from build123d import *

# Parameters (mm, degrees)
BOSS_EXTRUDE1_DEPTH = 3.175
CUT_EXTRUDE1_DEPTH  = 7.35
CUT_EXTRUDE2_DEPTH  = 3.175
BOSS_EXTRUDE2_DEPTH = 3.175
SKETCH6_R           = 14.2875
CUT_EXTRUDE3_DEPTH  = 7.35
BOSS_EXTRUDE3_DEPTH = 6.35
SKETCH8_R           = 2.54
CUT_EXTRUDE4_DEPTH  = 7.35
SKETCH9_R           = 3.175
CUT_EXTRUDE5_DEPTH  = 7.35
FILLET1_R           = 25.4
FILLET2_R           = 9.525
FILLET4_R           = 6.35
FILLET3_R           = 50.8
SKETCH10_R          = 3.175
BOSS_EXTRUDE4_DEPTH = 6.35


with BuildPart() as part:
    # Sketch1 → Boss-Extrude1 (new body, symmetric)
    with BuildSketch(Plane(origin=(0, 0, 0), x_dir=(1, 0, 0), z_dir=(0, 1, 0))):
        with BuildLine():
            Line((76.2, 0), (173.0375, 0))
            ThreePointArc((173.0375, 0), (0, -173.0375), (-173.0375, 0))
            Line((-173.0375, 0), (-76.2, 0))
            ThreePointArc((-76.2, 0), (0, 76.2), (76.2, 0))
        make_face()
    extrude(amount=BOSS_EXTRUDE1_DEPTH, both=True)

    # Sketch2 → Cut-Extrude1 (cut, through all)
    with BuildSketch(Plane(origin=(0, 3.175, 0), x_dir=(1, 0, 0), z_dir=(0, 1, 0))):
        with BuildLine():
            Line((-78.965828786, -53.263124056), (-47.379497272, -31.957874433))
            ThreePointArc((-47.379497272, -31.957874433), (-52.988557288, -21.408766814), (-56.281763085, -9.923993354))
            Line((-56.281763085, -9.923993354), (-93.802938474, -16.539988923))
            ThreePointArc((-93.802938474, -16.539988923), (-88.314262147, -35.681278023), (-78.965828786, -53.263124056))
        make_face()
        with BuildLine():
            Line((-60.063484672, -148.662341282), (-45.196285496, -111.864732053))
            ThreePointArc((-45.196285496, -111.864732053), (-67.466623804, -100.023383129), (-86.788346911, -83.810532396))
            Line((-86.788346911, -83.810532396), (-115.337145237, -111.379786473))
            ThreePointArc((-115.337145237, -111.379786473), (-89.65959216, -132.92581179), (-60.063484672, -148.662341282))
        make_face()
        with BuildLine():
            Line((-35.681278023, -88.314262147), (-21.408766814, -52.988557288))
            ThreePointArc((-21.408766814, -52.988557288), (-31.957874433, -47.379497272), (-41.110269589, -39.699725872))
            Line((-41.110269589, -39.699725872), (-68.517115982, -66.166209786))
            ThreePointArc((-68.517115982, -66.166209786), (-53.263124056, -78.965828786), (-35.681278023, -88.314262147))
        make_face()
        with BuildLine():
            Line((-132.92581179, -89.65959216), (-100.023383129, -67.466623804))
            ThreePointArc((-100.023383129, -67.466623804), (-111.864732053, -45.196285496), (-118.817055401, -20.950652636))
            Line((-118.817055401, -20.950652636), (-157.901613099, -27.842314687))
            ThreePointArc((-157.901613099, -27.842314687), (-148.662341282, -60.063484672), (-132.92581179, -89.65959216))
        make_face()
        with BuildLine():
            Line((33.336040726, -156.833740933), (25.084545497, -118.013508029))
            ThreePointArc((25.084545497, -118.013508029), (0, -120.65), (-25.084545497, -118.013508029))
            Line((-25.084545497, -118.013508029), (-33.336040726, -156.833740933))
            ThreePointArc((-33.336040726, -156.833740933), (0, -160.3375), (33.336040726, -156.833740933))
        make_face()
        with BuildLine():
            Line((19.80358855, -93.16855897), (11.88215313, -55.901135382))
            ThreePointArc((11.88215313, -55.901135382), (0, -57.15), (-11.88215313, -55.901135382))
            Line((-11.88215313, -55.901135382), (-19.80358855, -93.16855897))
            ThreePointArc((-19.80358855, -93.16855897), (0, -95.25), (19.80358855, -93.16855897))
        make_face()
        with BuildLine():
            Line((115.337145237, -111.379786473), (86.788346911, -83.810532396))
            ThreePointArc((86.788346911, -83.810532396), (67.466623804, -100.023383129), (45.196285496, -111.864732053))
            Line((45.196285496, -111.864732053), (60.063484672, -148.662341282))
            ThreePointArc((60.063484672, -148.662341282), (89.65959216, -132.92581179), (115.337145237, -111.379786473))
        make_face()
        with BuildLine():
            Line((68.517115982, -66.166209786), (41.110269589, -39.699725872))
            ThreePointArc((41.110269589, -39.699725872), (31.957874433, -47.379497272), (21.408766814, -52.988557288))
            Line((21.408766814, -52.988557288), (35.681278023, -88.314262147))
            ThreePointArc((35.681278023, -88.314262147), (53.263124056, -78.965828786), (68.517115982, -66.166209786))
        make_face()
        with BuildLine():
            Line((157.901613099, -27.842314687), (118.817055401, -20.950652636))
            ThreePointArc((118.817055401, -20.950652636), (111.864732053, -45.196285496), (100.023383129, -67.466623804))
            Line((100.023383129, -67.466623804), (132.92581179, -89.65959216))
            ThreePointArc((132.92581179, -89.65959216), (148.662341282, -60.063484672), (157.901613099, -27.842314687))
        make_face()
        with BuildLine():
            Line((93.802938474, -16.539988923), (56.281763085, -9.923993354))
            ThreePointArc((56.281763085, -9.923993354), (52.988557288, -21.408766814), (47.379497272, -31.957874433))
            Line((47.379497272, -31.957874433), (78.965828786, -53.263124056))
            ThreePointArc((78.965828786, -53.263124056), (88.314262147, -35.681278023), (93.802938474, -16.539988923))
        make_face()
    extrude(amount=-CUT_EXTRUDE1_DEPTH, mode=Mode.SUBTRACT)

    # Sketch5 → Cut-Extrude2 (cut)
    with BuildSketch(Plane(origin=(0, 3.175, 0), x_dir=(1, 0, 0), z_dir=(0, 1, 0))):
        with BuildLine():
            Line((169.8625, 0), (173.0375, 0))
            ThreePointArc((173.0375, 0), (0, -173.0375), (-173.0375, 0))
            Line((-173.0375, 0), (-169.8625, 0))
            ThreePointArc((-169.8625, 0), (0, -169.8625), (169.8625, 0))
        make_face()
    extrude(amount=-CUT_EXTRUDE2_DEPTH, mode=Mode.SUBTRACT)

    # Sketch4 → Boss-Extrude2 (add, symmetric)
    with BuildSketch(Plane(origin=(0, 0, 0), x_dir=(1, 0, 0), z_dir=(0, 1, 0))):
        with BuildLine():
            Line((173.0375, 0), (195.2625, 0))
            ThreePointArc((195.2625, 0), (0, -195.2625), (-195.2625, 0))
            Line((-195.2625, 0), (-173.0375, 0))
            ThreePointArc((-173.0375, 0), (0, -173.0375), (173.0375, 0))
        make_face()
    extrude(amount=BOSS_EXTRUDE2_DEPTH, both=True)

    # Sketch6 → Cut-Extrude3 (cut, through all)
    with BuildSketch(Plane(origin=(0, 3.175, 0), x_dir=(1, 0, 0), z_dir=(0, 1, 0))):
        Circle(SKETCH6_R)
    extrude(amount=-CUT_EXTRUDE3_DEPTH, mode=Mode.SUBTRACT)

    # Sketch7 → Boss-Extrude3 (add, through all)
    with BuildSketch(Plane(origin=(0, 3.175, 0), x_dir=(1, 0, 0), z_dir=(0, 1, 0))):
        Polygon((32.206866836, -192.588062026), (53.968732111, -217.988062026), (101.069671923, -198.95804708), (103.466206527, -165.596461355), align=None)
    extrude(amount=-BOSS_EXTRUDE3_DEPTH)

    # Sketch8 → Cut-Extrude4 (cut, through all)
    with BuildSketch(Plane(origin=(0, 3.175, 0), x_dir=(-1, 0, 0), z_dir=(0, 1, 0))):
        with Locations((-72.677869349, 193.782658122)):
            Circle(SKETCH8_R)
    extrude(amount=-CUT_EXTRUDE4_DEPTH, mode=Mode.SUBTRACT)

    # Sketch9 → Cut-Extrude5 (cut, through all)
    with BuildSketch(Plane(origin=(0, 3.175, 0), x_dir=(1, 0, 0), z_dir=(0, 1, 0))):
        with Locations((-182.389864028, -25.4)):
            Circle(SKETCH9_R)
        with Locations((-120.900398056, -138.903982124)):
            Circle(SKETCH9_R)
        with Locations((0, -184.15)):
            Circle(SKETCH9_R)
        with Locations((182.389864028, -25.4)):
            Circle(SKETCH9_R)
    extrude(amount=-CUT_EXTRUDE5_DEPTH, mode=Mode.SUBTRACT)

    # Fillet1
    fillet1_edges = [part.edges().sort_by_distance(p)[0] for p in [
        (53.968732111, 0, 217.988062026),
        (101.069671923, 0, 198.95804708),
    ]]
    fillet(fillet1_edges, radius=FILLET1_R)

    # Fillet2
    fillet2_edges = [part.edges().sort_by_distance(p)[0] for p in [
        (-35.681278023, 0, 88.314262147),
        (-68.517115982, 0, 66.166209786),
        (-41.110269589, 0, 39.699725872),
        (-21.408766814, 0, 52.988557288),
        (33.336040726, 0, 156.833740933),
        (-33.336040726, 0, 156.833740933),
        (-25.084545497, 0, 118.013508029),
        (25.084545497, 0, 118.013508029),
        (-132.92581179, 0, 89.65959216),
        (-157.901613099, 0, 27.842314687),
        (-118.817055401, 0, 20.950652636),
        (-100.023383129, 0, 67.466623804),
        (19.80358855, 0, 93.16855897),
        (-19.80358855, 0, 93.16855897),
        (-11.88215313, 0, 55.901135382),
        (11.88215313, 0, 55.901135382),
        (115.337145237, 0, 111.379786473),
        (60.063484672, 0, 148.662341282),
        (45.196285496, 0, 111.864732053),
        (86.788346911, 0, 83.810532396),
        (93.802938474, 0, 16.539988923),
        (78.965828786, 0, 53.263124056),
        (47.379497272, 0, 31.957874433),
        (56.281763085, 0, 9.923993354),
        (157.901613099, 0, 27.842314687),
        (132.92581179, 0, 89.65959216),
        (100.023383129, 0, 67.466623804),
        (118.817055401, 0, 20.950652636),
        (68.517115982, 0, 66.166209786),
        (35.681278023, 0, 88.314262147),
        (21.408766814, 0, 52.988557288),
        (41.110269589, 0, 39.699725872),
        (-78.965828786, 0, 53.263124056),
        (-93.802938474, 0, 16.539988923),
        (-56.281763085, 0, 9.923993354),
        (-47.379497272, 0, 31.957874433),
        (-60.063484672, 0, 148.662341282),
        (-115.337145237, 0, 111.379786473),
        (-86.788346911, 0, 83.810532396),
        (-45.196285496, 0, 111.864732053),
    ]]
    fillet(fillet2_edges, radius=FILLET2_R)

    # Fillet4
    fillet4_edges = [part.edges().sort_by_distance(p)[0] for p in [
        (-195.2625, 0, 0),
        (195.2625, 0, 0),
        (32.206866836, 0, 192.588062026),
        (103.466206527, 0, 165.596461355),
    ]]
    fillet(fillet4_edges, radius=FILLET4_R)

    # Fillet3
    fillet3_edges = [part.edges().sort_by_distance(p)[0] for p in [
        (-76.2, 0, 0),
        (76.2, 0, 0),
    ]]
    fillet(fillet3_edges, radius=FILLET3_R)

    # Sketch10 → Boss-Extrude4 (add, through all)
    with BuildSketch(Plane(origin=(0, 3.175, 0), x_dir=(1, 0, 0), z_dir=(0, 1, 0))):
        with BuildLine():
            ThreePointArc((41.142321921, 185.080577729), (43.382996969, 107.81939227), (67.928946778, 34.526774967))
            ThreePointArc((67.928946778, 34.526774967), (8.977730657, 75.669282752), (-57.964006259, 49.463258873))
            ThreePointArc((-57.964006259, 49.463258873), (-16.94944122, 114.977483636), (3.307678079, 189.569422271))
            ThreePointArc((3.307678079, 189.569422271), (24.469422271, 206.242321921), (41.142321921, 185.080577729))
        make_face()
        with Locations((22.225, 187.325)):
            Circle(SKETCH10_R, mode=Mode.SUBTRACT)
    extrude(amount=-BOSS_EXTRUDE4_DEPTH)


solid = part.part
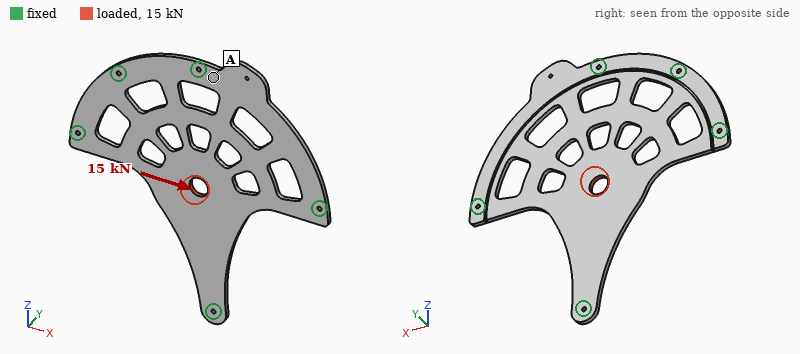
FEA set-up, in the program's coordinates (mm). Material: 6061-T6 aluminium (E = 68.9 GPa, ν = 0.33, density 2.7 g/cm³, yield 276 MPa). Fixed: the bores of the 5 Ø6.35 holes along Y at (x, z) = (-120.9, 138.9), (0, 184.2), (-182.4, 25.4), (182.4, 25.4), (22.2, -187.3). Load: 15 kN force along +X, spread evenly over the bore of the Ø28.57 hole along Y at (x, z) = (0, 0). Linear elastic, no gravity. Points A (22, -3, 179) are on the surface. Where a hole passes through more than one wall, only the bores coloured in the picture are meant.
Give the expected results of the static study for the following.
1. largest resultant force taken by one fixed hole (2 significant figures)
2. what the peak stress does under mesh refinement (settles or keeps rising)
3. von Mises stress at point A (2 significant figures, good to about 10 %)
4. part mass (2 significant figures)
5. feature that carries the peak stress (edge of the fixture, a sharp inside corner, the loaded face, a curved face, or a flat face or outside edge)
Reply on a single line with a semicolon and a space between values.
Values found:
5.5 kN; keeps rising; 9.2 MPa; 1.0 kg; a sharp inside corner
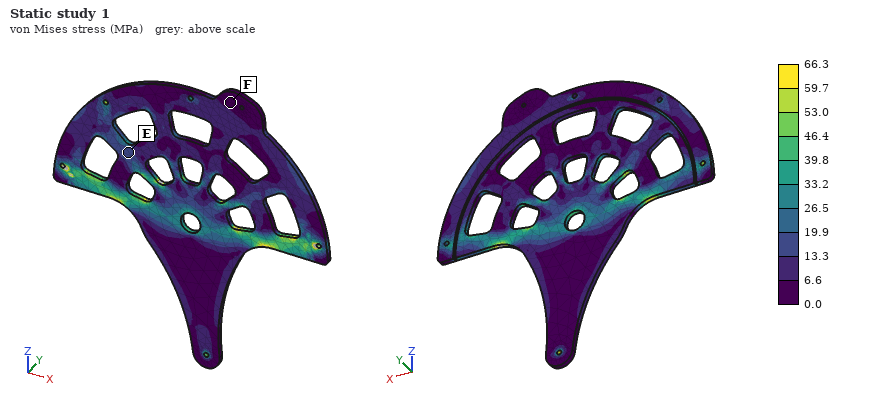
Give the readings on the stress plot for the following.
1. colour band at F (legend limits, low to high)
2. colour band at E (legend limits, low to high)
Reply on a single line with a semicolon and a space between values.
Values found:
0.0 to 6.6 MPa; 13.3 to 19.9 MPa
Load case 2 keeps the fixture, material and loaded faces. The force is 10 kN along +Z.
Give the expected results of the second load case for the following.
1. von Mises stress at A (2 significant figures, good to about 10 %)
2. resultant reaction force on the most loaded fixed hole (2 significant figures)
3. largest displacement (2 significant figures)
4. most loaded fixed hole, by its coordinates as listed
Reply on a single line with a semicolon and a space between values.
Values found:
11 MPa; 5.1 kN; 50 µm; (22.2, -187.3)
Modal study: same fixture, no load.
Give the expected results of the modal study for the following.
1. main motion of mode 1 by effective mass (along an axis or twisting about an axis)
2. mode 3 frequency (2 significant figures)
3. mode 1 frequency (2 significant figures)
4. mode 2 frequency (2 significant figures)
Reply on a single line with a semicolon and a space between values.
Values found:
along Y; 590 Hz; 260 Hz; 430 Hz
